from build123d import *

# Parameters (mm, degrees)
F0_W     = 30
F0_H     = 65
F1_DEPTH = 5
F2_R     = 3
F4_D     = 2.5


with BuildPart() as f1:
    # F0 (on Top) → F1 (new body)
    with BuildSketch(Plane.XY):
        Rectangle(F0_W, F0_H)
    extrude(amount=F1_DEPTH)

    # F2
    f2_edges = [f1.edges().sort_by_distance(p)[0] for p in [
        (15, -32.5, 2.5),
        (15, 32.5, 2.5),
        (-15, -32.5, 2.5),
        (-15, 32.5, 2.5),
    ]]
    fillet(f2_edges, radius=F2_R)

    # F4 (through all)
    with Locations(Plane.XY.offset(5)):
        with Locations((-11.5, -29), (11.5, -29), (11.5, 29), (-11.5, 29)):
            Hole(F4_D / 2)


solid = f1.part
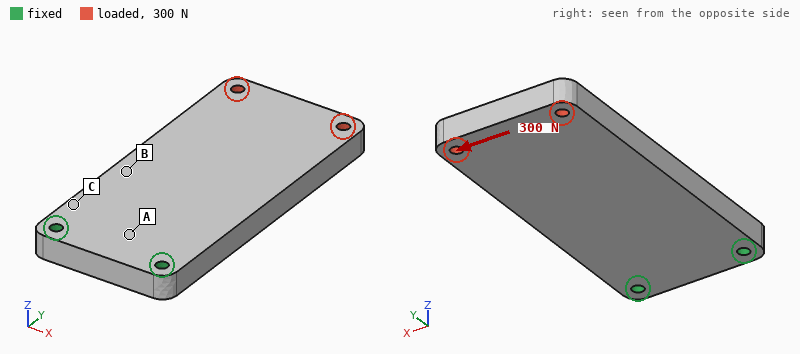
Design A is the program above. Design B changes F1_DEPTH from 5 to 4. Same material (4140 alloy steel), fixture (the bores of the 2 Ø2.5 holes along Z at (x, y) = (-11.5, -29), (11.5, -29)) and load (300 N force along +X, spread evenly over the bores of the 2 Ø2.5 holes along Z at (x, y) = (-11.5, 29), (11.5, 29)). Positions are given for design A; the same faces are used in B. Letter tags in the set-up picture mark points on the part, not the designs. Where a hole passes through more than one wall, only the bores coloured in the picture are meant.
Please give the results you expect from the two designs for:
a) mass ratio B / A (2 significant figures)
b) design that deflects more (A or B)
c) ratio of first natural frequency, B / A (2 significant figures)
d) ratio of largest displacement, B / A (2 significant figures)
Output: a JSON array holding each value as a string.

["0.80", "B", "0.81", "1.3"]
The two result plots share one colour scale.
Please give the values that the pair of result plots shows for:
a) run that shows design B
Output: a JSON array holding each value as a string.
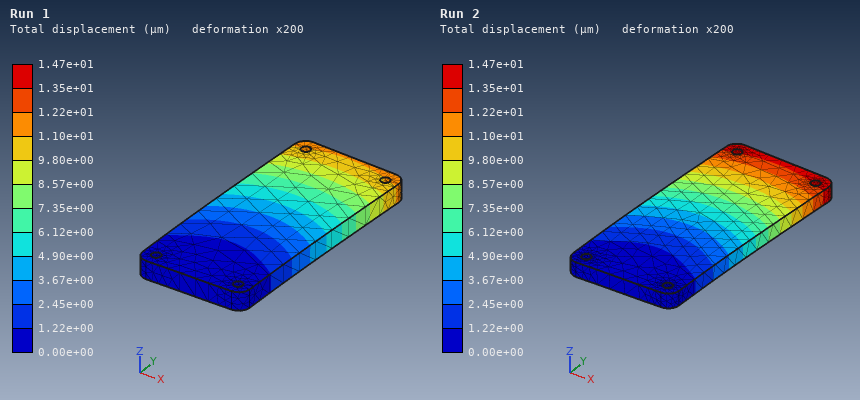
["Run 2"]
